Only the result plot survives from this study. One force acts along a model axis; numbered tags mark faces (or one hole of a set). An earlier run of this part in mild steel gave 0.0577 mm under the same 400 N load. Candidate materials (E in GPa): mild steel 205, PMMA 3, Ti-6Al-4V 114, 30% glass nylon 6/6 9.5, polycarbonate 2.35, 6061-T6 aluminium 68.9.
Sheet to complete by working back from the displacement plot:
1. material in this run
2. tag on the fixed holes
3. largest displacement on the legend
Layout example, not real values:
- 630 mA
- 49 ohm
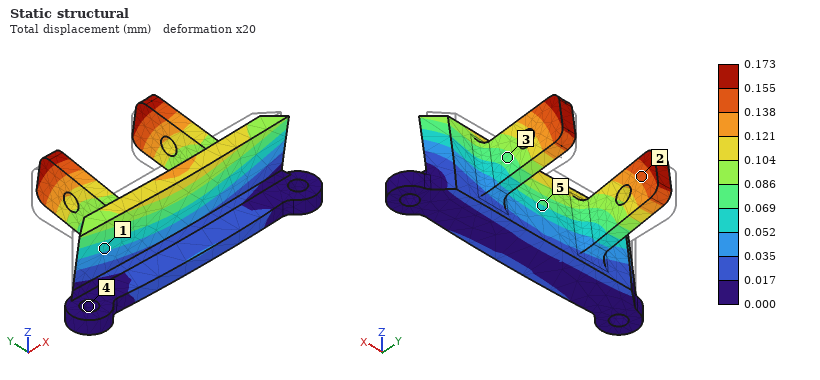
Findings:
- 6061-T6 aluminium
- 4
- 0.173 mm
